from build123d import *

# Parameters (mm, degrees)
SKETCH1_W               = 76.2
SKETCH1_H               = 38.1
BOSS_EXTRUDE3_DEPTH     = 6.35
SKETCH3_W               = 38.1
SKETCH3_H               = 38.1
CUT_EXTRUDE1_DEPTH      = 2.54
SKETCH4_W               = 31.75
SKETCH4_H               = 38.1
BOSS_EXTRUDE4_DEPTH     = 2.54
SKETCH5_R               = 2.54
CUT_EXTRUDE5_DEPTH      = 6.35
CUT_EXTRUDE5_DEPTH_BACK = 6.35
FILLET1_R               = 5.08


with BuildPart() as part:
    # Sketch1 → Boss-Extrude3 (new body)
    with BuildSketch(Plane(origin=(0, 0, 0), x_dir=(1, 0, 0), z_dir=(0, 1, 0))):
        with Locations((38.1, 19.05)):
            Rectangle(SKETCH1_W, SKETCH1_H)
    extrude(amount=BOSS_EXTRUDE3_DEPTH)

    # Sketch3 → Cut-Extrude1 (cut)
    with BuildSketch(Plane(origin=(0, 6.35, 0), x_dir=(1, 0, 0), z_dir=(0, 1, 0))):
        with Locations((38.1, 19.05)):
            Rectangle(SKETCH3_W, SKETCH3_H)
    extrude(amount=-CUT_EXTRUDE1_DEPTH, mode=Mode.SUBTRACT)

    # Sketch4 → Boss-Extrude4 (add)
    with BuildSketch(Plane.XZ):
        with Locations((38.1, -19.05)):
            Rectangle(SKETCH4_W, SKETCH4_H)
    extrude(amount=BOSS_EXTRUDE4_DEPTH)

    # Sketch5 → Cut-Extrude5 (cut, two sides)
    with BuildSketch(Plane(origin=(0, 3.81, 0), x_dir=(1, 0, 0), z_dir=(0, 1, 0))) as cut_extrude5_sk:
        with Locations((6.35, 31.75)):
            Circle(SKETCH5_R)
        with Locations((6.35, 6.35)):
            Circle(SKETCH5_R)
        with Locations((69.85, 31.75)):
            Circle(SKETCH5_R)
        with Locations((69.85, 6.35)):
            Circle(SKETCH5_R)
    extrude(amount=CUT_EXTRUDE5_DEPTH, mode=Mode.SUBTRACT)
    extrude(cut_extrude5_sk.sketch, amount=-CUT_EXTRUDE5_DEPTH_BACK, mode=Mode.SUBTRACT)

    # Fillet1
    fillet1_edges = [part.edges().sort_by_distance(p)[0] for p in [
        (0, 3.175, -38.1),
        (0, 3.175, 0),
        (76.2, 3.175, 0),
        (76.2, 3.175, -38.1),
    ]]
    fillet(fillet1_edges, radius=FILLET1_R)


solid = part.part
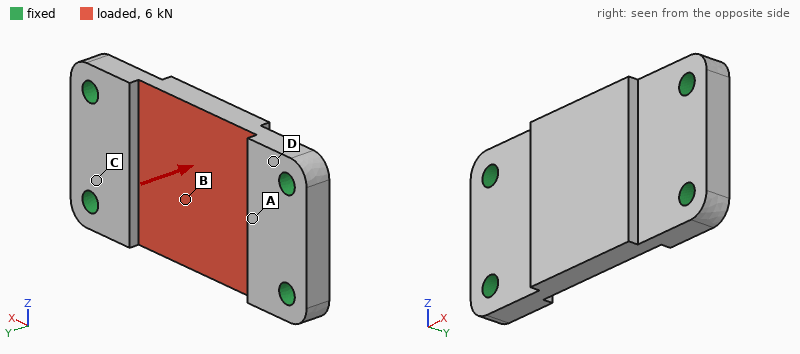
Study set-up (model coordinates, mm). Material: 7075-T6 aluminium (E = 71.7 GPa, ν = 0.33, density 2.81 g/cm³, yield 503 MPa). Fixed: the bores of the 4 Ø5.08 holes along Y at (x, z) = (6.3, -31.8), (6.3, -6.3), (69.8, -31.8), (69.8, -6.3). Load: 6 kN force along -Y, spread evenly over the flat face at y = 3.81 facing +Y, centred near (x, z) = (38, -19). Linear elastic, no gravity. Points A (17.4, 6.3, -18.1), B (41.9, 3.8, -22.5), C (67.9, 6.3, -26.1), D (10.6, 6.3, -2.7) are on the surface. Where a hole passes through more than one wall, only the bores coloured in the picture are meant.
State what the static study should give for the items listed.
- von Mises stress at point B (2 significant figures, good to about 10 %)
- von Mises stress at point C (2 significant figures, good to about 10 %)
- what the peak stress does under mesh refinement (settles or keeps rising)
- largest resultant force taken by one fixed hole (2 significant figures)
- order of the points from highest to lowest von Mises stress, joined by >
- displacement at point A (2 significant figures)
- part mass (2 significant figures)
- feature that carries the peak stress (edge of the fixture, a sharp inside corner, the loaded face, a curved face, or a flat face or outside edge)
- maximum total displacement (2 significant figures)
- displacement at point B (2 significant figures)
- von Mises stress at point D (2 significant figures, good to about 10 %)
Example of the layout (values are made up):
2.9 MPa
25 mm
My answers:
46 MPa
73 MPa
keeps rising
2.6 kN
D > C > B > A
38 µm
48 g
edge of the fixture
98 µm
88 µm
110 MPa
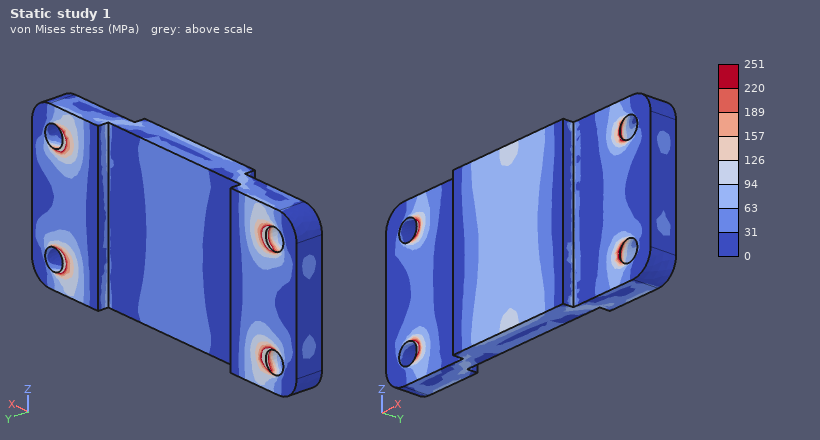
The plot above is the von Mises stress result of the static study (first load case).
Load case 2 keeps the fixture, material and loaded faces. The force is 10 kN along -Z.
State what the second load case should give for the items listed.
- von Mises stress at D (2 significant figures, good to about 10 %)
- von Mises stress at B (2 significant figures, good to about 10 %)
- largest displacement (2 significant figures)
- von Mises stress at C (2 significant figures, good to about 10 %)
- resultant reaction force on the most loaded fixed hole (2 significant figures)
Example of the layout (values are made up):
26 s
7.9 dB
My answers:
24 MPa
21 MPa
42 µm
42 MPa
3.2 kN
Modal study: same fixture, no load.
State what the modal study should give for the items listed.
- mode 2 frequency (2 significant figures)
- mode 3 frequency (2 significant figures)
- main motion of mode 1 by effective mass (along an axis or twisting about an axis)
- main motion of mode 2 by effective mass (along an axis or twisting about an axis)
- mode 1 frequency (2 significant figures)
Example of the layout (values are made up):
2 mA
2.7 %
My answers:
11 kHz
17 kHz
along Y
twisting about X
8600 Hz
